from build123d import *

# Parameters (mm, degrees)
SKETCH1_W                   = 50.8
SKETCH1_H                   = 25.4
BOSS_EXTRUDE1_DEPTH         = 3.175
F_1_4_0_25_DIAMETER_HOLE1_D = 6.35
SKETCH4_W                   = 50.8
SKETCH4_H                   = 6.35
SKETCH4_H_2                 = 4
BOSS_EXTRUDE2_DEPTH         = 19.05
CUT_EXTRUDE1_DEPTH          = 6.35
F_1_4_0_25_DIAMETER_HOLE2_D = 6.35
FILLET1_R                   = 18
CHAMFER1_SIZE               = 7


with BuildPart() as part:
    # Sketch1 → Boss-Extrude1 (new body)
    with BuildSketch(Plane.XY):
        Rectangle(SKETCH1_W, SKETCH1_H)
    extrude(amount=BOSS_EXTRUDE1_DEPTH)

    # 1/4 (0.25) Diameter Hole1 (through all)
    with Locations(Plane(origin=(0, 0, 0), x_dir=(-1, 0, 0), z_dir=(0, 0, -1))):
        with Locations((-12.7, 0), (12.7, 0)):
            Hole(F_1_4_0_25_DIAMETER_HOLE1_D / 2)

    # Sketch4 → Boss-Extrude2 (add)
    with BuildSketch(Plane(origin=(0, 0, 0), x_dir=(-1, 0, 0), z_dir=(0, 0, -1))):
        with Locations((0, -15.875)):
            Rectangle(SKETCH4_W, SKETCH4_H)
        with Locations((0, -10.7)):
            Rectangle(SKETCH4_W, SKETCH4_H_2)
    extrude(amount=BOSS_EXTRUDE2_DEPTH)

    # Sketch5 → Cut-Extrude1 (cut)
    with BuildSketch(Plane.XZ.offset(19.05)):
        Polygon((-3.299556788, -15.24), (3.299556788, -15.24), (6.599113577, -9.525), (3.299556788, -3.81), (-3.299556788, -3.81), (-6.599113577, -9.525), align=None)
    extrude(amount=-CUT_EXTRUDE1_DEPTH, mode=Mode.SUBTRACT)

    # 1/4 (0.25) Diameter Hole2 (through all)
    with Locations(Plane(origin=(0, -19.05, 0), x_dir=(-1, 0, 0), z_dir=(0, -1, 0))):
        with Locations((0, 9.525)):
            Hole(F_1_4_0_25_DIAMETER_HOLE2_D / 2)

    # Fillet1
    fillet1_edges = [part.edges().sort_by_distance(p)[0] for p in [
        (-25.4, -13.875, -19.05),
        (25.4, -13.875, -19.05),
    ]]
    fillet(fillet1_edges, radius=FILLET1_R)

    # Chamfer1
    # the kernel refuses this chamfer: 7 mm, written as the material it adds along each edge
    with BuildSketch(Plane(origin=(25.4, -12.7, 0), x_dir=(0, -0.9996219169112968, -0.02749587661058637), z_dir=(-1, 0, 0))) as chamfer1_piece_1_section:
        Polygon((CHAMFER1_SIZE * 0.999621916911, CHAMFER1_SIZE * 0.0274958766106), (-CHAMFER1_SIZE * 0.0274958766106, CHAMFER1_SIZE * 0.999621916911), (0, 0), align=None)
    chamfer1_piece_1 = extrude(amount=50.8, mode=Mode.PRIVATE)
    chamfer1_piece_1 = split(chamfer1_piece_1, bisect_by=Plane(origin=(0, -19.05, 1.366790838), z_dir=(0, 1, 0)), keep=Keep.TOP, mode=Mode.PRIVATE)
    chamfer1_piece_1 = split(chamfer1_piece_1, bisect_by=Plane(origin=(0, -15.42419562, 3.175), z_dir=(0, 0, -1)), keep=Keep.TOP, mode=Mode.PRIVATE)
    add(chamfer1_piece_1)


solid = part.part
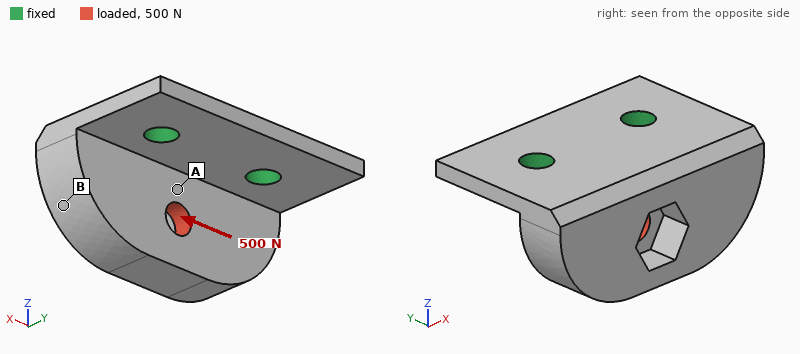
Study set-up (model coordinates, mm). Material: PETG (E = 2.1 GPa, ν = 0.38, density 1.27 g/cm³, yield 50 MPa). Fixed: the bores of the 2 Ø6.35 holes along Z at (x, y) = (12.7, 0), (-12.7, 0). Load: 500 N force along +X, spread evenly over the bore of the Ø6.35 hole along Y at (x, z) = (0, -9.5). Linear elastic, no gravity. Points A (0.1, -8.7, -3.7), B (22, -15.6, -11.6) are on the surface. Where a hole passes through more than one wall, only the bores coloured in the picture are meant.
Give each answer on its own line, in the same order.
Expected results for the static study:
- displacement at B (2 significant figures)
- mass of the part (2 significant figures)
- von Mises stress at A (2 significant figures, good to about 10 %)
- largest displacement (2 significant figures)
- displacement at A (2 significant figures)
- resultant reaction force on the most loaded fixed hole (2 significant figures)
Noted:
0.37 mm
16 g
12 MPa
0.38 mm
0.13 mm
350 N
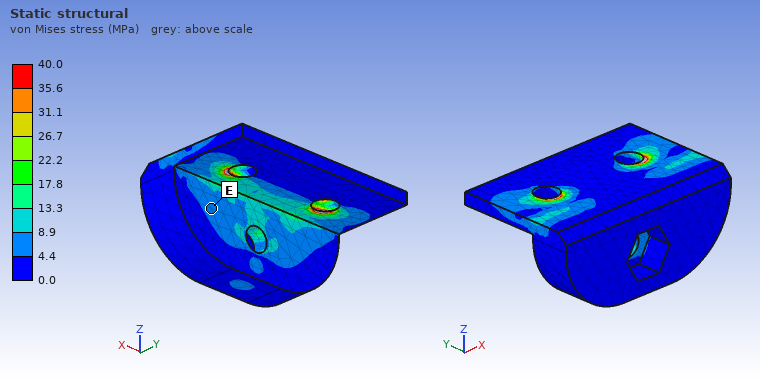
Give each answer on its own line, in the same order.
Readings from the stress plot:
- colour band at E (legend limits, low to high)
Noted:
4.4 to 8.9 MPa
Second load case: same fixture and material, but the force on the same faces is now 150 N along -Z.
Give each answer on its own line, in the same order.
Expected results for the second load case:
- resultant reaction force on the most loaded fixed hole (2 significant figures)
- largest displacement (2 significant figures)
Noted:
75 N
0.56 mm
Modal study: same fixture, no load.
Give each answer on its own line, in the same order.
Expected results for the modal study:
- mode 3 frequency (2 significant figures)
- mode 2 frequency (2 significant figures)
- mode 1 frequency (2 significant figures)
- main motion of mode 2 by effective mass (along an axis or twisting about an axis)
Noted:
3000 Hz
1700 Hz
630 Hz
along X
